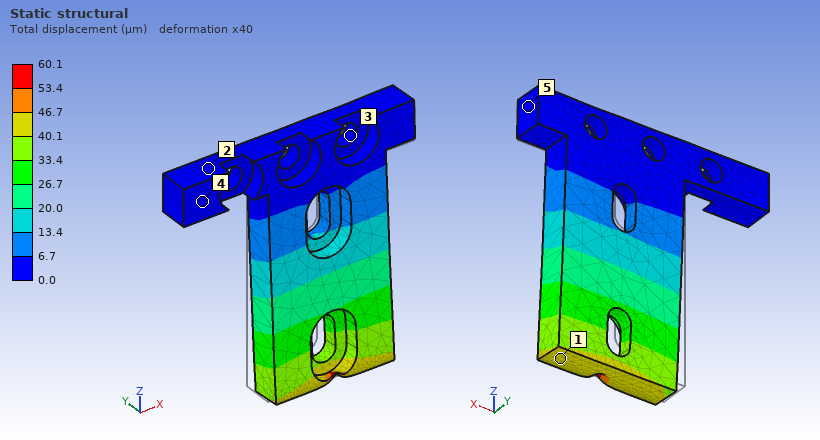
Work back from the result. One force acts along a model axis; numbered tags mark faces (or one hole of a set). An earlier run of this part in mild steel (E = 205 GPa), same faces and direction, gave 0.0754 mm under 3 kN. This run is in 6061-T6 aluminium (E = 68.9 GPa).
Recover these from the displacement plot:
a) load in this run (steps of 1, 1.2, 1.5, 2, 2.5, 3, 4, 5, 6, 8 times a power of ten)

800 N
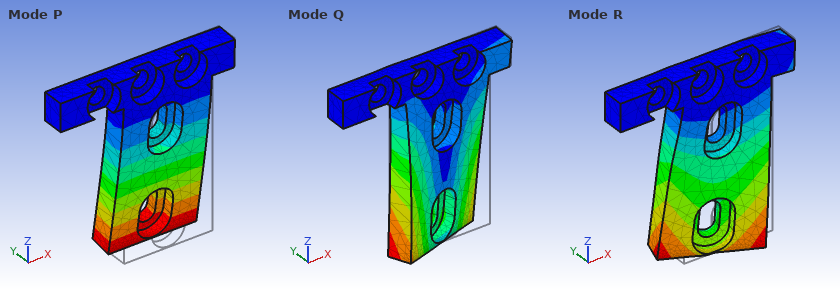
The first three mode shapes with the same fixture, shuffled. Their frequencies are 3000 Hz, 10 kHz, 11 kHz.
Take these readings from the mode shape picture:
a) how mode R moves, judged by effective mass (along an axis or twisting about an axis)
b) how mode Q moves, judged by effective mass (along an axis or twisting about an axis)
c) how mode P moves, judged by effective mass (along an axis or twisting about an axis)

along X
along X
along Y
